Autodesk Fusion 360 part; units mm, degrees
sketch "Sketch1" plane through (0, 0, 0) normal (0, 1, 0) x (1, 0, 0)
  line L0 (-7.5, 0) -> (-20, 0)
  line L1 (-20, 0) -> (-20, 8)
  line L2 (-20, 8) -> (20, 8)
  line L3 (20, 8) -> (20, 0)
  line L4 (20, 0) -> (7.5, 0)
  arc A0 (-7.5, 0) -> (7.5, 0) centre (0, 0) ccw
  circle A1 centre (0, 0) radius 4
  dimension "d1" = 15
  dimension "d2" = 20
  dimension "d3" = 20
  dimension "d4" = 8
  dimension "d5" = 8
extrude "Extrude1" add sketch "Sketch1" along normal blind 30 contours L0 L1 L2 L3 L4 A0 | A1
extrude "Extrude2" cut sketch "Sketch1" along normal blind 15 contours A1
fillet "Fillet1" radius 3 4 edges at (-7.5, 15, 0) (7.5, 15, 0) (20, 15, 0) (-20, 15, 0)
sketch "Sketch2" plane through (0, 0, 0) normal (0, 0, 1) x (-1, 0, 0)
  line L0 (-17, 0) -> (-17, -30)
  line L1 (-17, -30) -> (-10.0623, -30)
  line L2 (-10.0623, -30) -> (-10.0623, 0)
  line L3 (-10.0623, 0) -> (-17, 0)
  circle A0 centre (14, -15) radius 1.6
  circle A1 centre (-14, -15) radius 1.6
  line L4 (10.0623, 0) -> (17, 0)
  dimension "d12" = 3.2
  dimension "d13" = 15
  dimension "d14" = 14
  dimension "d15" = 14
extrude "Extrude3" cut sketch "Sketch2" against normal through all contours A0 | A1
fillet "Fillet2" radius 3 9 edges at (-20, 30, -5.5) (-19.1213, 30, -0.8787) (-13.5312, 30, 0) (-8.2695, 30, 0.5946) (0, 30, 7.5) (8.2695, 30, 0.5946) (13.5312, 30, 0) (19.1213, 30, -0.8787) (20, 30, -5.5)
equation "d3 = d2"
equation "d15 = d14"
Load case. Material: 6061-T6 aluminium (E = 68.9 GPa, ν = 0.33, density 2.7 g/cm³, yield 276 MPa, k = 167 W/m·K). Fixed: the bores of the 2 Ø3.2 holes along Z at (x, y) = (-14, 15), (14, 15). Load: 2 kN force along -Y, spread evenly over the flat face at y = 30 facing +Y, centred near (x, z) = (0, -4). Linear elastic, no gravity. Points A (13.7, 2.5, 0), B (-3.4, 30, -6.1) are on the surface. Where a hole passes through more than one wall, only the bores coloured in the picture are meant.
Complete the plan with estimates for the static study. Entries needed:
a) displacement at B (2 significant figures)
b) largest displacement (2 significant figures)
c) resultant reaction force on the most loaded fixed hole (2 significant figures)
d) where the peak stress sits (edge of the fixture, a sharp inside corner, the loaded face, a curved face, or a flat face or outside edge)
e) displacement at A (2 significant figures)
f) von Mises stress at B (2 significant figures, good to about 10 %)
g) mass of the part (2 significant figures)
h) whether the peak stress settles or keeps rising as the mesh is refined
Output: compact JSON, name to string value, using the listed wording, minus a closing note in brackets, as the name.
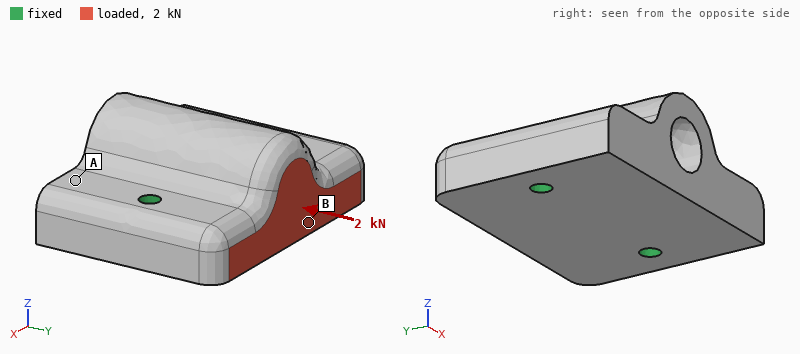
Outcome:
{"displacement at B": "3.0 µm", "largest displacement": "3.2 µm", "resultant reaction force on the most loaded fixed hole": "1.0 kN", "where the peak stress sits": "edge of the fixture", "displacement at A": "0.96 µm", "von Mises stress at B": "8.0 MPa", "mass of the part": "30 g", "whether the peak stress settles or keeps rising as the mesh is refined": "keeps rising"}
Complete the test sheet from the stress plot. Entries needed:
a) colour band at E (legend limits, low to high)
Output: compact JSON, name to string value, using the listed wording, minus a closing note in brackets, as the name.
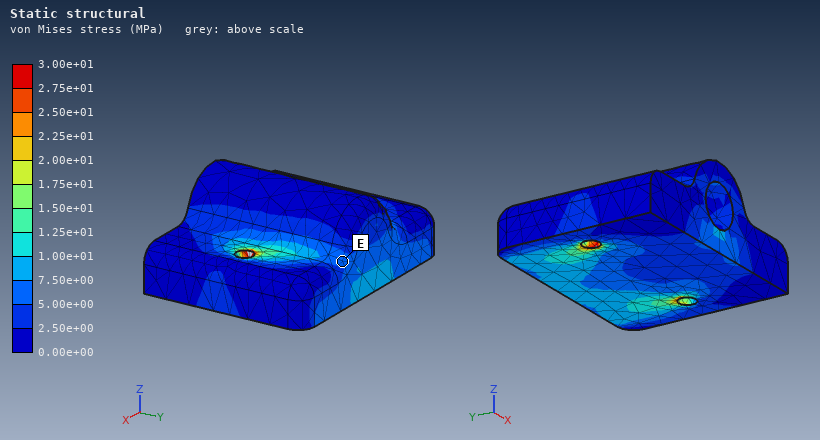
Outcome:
{"colour band at E": "5.00e+00 to 7.50e+00 MPa"}
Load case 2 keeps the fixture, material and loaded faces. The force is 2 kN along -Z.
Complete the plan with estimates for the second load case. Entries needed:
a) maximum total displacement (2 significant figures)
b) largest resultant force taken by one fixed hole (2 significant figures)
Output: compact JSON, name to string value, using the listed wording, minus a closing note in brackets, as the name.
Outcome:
{"maximum total displacement": "37 µm", "largest resultant force taken by one fixed hole": "1.0 kN"}
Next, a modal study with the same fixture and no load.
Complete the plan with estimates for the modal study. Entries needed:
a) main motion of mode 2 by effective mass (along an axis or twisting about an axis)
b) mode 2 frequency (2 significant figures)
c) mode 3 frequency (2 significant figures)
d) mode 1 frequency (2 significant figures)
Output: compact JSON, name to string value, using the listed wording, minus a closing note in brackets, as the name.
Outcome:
{"main motion of mode 2 by effective mass": "along Z", "mode 2 frequency": "22 kHz", "mode 3 frequency": "31 kHz", "mode 1 frequency": "14 kHz"}
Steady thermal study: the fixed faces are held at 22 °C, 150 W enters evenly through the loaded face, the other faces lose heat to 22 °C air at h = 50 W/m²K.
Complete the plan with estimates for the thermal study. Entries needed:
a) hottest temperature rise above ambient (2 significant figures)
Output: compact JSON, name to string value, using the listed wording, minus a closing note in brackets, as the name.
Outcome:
{"hottest temperature rise above ambient": "55 K"}
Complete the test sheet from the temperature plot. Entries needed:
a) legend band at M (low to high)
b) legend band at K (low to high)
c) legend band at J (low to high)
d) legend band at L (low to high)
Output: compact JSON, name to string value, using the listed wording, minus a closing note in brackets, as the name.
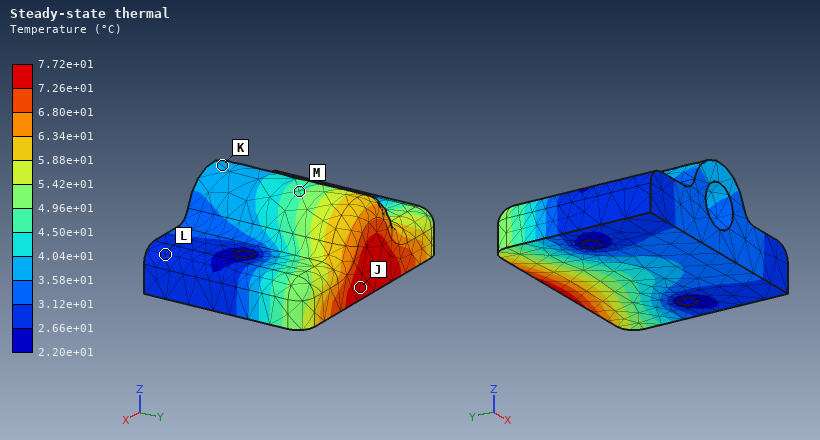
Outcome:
{"legend band at M": "4.50e+01 to 4.96e+01 °C", "legend band at K": "3.58e+01 to 4.04e+01 °C", "legend band at J": "7.26e+01 to 7.72e+01 °C", "legend band at L": "2.66e+01 to 3.12e+01 °C"}
